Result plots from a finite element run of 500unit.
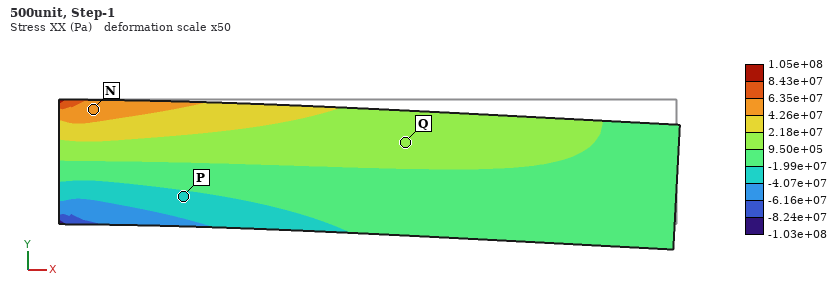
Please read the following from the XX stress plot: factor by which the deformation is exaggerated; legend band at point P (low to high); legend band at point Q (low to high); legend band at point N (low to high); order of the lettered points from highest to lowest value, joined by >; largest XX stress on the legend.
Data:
50
-4.07e+07 to -1.99e+07 Pa
9.50e+05 to 2.18e+07 Pa
4.26e+07 to 6.35e+07 Pa
N > Q > P
1.05e+08 Pa
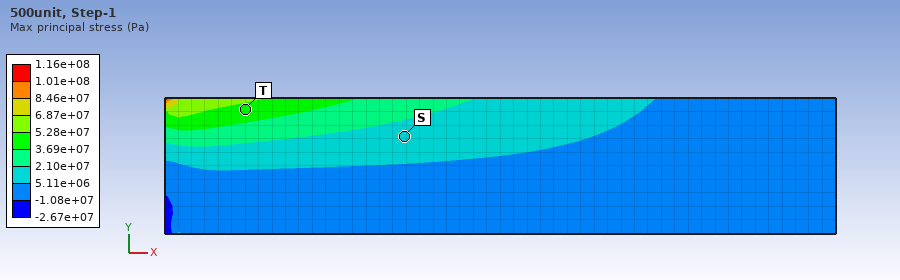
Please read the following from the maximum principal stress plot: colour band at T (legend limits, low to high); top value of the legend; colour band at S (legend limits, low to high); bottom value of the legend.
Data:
3.69e+07 to 5.28e+07 Pa
1.16e+08 Pa
5.11e+06 to 2.10e+07 Pa
-2.67e+07 Pa
